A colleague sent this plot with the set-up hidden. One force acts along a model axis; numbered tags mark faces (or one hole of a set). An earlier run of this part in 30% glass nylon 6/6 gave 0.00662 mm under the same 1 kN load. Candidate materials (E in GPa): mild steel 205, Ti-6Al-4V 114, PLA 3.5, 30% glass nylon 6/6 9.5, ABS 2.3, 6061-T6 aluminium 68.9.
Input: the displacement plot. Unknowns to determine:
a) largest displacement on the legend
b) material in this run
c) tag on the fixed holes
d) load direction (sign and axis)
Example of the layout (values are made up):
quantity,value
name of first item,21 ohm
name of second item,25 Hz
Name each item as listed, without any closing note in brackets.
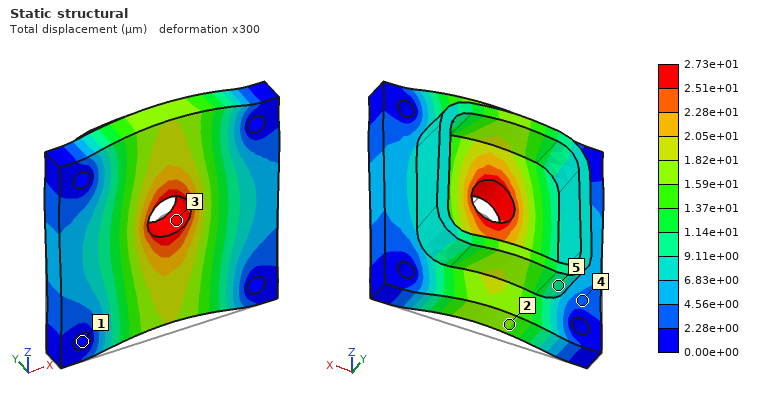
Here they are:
quantity,value
largest displacement on the legend,2.73e+01 µm
material in this run,ABS
tag on the fixed holes,1
load direction,+Z
